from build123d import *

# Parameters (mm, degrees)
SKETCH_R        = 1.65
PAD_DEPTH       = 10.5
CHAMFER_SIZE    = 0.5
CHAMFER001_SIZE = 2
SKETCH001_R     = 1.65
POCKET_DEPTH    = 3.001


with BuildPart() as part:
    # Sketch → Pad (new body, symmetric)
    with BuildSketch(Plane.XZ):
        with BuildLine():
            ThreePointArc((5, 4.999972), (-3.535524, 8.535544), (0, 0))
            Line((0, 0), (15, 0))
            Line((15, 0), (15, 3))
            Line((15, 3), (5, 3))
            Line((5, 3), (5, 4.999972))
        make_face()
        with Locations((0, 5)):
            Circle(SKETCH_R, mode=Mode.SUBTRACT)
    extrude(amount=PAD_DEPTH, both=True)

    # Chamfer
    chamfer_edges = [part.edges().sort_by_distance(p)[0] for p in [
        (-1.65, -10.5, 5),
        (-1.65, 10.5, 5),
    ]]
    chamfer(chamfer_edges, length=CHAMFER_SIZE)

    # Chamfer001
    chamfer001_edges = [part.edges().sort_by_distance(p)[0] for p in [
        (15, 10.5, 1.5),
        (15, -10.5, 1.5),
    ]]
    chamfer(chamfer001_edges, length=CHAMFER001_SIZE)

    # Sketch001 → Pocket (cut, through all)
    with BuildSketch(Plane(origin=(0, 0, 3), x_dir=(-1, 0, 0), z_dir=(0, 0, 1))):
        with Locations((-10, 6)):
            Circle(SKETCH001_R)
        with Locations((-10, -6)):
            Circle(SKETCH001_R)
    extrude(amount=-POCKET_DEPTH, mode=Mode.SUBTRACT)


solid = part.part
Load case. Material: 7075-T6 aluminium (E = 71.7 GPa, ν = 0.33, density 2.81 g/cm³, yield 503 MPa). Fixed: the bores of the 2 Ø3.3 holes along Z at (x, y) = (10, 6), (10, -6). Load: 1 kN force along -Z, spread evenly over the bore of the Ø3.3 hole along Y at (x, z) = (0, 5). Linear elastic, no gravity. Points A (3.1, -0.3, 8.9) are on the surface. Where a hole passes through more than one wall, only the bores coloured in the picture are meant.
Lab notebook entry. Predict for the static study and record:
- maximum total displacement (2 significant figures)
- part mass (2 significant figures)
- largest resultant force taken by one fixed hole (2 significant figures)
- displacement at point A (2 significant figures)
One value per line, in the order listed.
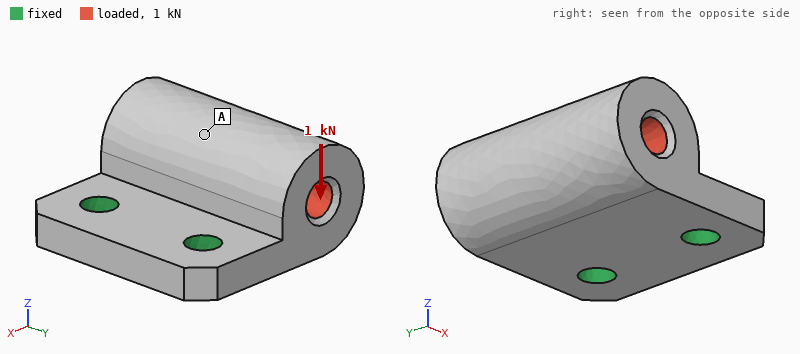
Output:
0.14 mm
6.0 g
500 N
0.092 mm
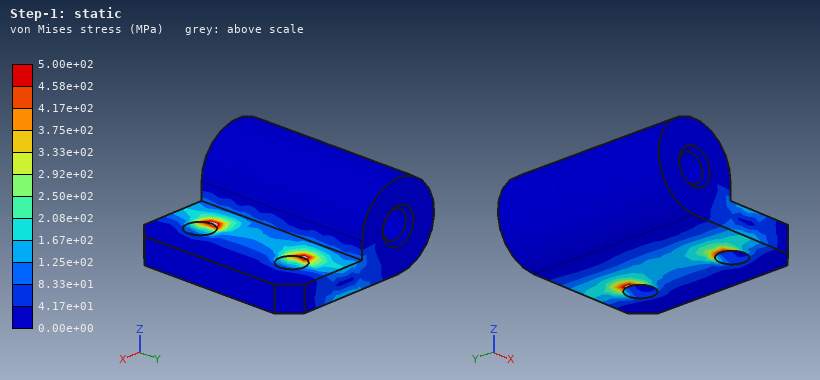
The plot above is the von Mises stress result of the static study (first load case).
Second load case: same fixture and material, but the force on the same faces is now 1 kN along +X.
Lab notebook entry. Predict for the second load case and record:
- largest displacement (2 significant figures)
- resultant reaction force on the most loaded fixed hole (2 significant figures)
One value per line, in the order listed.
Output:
72 µm
510 N
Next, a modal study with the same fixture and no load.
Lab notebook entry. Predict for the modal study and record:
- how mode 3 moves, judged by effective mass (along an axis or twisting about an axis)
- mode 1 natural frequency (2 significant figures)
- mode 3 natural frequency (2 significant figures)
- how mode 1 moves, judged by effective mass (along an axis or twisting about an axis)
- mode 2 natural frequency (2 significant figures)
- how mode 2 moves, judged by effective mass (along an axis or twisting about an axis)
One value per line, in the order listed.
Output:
along Y
7100 Hz
27 kHz
along Z
19 kHz
along Y
